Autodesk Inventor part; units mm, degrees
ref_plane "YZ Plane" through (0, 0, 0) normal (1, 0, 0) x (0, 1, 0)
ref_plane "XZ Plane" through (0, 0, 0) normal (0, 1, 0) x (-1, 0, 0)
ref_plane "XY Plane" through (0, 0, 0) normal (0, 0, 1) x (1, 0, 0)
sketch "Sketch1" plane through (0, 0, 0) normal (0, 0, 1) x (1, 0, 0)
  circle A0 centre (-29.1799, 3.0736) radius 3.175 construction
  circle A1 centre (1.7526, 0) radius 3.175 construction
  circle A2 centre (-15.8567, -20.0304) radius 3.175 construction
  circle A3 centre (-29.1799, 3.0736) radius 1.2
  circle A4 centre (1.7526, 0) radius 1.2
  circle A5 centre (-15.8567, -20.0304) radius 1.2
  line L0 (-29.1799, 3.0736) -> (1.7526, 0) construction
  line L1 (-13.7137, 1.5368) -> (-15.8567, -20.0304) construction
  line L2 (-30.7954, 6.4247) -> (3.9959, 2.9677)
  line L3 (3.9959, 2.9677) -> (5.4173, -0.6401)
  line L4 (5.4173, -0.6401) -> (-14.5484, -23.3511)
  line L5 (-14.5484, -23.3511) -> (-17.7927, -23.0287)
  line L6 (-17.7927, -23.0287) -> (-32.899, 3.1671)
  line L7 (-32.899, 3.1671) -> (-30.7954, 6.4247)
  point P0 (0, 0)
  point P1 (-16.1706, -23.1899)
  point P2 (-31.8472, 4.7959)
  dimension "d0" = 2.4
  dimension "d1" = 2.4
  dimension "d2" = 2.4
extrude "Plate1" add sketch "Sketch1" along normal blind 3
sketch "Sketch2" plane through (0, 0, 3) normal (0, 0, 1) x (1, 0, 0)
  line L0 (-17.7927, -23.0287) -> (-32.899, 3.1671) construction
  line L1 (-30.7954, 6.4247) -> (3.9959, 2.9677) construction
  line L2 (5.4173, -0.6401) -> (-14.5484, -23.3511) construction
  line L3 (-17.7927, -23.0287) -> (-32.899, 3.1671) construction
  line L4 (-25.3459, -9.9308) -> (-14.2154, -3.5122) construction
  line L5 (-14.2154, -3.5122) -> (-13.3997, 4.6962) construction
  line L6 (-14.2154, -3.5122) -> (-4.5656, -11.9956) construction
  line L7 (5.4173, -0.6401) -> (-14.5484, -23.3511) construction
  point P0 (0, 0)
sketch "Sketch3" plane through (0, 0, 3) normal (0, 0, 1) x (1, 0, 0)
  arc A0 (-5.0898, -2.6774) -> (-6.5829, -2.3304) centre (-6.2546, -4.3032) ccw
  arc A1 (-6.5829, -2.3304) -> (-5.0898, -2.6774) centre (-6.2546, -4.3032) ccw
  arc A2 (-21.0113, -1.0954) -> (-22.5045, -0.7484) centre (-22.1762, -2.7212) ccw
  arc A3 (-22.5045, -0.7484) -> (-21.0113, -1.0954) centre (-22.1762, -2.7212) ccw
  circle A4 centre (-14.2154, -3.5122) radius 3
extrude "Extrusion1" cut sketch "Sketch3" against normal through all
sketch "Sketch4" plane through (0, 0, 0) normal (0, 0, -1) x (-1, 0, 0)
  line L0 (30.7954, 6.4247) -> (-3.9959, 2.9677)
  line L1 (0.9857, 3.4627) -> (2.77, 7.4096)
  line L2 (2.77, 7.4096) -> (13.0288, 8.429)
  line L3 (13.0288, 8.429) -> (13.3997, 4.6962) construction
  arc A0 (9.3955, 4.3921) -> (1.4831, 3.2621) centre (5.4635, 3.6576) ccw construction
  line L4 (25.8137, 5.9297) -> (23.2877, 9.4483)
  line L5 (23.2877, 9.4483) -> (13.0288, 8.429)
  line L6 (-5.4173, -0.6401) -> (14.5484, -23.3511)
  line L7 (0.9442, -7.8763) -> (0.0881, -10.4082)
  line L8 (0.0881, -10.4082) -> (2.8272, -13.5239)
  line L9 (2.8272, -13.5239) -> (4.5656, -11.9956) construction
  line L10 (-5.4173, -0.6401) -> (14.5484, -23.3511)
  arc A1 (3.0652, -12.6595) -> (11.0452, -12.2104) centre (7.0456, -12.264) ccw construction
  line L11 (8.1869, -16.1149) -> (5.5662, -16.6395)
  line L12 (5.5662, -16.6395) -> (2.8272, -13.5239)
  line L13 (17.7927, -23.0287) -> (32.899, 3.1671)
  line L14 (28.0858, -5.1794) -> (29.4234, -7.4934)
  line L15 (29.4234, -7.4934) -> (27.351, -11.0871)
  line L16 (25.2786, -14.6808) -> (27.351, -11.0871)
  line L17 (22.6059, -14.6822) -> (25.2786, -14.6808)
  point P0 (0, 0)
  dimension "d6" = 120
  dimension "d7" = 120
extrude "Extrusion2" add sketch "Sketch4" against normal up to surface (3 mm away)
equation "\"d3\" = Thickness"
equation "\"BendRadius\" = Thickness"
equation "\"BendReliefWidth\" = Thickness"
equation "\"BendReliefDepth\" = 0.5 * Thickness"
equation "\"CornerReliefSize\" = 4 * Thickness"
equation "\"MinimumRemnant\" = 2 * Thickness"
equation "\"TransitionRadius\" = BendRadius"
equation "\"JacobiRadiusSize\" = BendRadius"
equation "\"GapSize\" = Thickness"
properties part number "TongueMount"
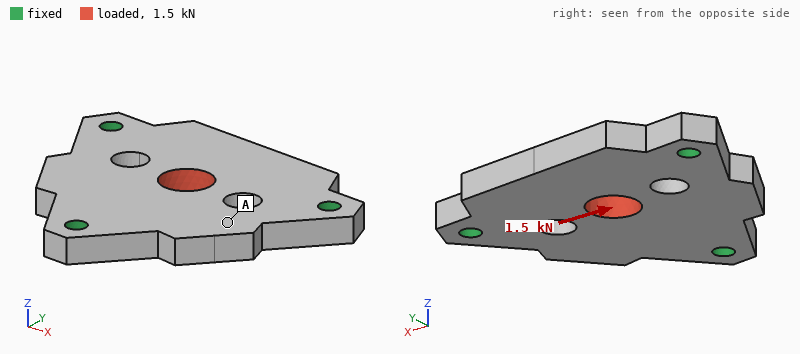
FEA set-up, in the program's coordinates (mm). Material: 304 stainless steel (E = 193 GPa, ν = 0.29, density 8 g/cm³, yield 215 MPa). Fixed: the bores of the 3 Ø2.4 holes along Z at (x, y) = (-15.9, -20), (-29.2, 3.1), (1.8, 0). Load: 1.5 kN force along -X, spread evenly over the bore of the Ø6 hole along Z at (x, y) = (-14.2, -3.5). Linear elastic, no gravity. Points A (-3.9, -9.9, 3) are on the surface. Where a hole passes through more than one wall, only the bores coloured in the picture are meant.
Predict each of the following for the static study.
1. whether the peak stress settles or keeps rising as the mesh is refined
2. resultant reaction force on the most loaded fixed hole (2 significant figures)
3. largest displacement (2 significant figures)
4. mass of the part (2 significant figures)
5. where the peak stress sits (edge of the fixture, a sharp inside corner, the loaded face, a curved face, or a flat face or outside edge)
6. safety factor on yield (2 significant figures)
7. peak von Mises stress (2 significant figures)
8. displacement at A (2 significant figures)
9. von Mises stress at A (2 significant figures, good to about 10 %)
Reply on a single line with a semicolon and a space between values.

settles; 610 N; 3.0 µm; 17 g; a curved face; 2.7; 80 MPa; 1.9 µm; 11 MPa
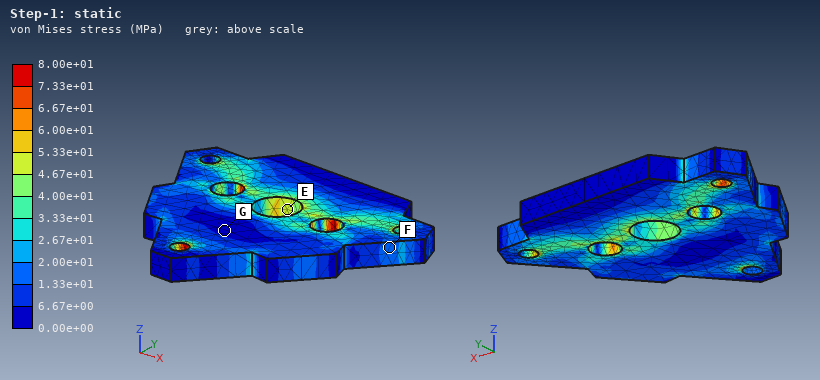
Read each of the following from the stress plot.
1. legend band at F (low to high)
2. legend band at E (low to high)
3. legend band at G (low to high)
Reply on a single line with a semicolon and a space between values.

1.33e+01 to 2.00e+01 MPa; 4.67e+01 to 5.33e+01 MPa; 0.00e+00 to 6.67e+00 MPa
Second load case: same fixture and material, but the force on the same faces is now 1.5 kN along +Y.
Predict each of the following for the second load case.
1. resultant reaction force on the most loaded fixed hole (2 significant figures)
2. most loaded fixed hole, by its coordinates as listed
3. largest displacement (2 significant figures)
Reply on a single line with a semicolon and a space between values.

790 N; (-15.9, -20); 3.5 µm
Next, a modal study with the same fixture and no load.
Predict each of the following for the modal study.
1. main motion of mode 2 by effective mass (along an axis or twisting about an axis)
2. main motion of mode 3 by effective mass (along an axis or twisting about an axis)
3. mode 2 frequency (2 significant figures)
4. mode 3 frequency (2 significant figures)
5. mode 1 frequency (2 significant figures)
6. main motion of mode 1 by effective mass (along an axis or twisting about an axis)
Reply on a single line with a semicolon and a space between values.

along Z; twisting about Y; 18 kHz; 20 kHz; 13 kHz; along Z
